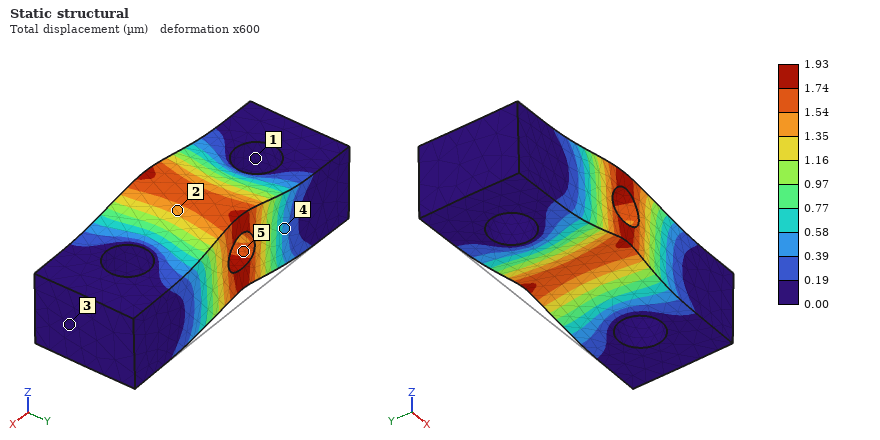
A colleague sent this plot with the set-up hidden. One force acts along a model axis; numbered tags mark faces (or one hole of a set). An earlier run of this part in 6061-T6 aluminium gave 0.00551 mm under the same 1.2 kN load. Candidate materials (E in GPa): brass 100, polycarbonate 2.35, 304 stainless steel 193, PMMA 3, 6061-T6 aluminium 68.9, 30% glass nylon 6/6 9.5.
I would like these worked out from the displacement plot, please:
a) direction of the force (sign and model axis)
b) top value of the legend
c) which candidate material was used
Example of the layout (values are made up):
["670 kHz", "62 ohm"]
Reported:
["+Z", "1.93 µm", "304 stainless steel"]
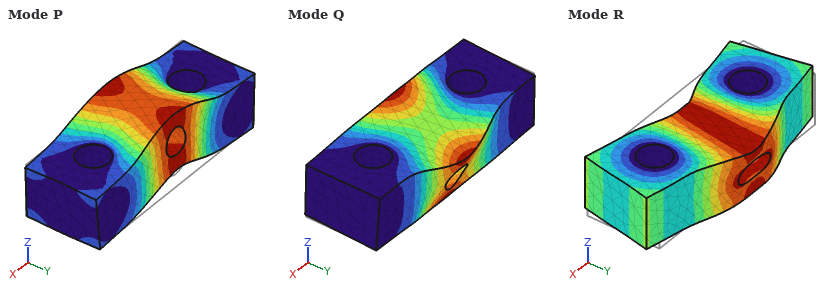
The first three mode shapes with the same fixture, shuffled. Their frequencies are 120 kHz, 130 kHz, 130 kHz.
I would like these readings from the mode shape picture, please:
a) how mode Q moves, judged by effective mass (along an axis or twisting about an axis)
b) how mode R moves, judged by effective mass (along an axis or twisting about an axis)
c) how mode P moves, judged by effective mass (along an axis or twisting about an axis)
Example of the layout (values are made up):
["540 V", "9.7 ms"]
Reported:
["twisting about X", "along Y", "along Z"]
